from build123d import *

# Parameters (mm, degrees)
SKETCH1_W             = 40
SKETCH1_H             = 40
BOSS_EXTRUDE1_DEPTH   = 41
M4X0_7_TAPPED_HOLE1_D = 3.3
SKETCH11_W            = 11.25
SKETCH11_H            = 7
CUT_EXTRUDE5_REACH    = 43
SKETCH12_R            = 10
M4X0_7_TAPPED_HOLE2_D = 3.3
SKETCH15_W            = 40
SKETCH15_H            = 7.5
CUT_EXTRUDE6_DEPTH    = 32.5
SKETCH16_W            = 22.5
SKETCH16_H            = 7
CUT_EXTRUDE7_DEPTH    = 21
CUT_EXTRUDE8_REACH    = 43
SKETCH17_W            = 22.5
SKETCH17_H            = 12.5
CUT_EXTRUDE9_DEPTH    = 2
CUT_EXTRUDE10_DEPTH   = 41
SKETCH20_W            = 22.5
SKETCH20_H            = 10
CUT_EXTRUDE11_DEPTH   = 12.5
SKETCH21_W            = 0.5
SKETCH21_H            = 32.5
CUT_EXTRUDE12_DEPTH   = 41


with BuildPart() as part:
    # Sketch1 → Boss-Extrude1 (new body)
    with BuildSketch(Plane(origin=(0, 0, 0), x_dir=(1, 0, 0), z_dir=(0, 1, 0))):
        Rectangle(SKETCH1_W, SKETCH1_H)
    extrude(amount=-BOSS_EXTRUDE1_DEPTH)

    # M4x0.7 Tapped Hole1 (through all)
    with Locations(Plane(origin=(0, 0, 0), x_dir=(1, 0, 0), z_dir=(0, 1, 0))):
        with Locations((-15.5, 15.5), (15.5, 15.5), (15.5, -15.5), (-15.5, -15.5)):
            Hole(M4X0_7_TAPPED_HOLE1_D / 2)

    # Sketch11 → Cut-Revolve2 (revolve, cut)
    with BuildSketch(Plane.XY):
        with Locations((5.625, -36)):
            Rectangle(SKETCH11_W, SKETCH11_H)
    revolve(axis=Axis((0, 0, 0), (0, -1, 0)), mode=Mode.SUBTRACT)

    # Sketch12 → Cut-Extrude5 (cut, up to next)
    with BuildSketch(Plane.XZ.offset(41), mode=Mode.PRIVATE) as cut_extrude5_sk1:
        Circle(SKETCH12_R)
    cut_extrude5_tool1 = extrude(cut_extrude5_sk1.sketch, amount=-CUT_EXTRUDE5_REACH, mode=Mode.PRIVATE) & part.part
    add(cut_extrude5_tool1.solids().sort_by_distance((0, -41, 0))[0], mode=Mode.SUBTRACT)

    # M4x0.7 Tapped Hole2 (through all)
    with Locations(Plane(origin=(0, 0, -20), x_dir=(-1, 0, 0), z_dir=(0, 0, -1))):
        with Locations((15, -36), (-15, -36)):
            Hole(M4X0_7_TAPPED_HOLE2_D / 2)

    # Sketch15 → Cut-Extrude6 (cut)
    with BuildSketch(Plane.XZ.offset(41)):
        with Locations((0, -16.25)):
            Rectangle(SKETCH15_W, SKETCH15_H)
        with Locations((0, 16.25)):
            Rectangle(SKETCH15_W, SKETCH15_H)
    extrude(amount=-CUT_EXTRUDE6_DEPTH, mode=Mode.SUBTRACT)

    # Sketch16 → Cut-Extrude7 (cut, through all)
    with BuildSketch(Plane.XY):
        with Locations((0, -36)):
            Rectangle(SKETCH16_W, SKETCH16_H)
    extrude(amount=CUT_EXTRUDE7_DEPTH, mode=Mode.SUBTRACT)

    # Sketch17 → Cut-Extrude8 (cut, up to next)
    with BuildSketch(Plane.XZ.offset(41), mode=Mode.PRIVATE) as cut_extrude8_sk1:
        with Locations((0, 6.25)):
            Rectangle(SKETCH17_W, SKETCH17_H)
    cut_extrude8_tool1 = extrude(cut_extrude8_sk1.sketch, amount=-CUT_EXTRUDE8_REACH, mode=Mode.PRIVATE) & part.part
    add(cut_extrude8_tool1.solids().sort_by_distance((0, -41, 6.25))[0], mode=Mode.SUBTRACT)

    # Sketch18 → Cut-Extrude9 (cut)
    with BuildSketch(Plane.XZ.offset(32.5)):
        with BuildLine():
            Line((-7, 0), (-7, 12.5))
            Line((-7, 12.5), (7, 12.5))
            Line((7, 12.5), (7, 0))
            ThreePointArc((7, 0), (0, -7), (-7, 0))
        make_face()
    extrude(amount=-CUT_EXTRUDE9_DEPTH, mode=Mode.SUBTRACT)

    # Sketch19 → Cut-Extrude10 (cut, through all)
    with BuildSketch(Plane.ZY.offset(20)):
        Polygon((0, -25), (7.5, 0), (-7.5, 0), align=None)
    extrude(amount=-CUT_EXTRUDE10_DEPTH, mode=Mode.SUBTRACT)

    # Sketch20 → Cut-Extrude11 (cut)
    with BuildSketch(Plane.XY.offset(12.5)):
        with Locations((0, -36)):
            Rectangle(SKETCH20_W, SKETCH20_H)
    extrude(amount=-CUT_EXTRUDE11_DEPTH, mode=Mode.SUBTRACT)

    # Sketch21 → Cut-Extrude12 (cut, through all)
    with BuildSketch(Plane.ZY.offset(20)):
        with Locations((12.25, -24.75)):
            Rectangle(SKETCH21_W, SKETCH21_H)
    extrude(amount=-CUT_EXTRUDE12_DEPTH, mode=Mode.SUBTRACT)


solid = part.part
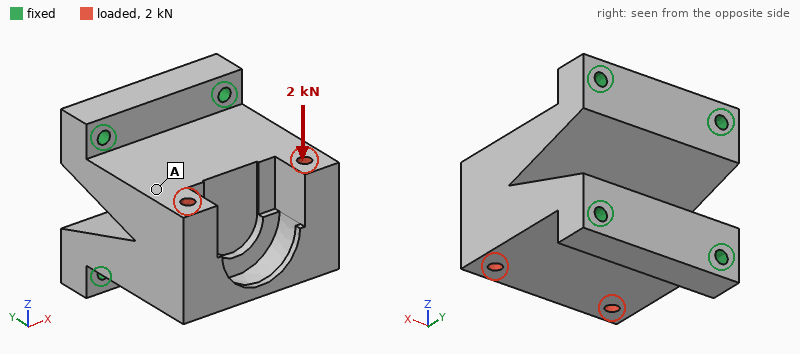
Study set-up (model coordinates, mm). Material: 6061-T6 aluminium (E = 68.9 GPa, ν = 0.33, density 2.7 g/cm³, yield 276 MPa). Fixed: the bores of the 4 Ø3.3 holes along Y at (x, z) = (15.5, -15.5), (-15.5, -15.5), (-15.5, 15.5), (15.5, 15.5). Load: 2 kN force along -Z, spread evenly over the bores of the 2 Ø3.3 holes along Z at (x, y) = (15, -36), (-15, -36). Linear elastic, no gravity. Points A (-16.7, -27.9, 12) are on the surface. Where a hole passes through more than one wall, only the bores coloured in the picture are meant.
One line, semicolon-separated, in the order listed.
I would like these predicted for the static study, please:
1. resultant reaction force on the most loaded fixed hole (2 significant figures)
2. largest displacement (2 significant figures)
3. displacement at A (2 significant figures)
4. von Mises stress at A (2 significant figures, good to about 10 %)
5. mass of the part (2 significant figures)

1.3 kN; 22 µm; 14 µm; 5.8 MPa; 88 g
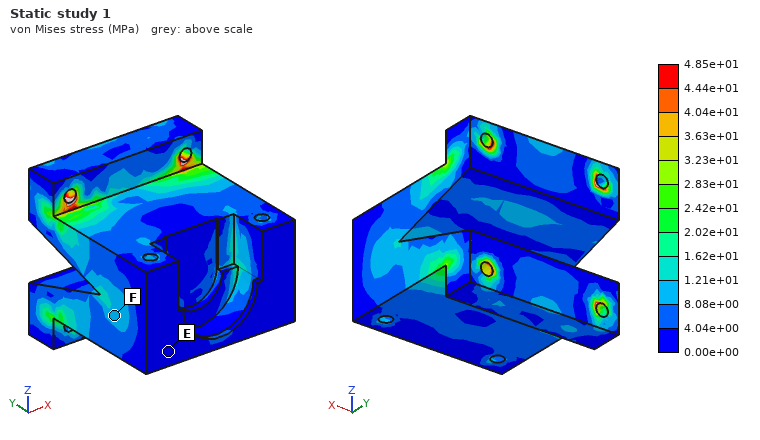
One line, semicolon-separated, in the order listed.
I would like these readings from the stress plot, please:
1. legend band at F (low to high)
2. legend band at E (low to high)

8.08e+00 to 1.21e+01 MPa; 0.00e+00 to 4.04e+00 MPa
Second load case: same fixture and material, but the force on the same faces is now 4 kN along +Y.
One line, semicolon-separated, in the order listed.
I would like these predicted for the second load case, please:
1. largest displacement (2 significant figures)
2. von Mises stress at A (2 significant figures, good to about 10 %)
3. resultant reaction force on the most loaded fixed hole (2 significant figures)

7.8 µm; 7.4 MPa; 1.1 kN
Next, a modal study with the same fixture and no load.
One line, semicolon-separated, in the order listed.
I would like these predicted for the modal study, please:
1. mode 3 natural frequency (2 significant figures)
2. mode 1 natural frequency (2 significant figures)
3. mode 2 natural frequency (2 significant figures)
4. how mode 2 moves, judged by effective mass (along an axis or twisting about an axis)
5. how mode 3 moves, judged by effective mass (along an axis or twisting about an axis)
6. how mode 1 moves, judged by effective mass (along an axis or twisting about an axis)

15 kHz; 10000 Hz; 10 kHz; along X; twisting about Y; along Z
